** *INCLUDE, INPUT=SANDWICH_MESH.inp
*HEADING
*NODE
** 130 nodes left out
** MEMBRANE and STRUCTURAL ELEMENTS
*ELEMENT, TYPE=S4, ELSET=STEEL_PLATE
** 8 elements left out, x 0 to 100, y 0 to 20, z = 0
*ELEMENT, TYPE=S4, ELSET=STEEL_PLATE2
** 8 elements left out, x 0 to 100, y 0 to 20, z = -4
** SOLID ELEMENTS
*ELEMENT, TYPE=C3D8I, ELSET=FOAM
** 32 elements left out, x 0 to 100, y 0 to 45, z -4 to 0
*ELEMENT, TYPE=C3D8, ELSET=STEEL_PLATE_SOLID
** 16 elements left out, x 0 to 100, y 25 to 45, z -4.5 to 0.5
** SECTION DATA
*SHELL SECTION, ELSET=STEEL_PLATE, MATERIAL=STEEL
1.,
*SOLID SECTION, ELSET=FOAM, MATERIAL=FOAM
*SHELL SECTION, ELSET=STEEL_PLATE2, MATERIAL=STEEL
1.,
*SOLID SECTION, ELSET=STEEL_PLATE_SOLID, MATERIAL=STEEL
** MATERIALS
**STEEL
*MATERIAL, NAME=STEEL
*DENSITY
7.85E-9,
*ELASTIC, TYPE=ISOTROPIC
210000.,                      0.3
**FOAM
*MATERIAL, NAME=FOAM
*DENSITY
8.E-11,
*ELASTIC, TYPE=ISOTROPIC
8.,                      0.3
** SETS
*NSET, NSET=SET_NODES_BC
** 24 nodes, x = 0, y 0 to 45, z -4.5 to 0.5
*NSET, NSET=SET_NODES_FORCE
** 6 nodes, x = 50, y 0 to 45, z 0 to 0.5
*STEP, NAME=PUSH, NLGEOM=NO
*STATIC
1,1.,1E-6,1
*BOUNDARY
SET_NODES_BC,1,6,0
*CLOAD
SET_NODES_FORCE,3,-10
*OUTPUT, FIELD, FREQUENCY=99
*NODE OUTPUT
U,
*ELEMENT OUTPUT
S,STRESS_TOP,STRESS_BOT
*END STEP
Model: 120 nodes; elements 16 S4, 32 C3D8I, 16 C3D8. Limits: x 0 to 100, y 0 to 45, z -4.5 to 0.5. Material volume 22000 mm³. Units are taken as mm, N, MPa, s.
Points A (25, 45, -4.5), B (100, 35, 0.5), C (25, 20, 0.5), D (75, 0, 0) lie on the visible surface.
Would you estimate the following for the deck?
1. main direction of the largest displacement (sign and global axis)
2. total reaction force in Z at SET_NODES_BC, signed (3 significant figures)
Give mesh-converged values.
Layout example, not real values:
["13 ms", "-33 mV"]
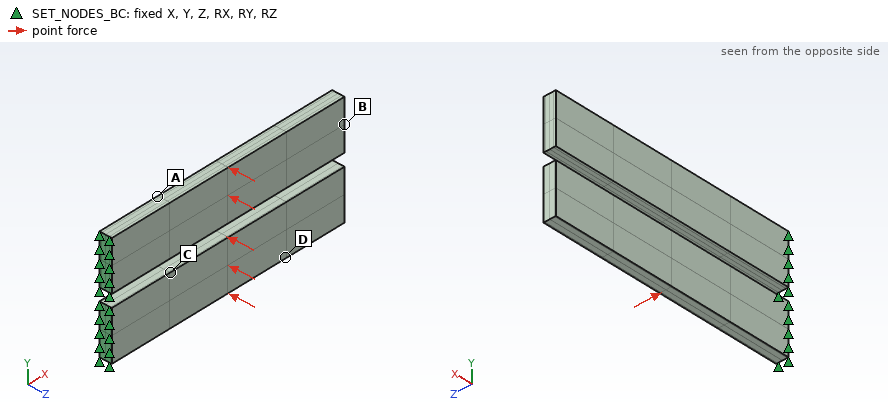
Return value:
["-Z", "60.0 N"]
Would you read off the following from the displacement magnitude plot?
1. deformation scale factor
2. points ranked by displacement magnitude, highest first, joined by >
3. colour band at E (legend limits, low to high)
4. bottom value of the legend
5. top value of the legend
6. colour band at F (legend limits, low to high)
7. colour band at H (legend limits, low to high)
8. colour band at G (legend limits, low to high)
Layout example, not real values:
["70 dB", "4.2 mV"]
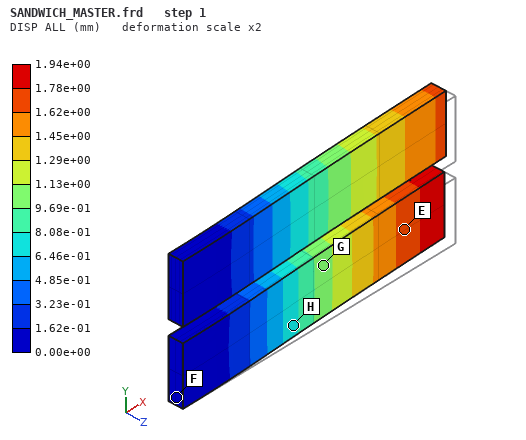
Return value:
["2", "E > G > H > F", "1.62e+00 to 1.78e+00 mm", "0.00e+00 mm", "1.94e+00 mm", "0.00e+00 to 1.62e-01 mm", "6.46e-01 to 8.08e-01 mm", "9.69e-01 to 1.13e+00 mm"]
